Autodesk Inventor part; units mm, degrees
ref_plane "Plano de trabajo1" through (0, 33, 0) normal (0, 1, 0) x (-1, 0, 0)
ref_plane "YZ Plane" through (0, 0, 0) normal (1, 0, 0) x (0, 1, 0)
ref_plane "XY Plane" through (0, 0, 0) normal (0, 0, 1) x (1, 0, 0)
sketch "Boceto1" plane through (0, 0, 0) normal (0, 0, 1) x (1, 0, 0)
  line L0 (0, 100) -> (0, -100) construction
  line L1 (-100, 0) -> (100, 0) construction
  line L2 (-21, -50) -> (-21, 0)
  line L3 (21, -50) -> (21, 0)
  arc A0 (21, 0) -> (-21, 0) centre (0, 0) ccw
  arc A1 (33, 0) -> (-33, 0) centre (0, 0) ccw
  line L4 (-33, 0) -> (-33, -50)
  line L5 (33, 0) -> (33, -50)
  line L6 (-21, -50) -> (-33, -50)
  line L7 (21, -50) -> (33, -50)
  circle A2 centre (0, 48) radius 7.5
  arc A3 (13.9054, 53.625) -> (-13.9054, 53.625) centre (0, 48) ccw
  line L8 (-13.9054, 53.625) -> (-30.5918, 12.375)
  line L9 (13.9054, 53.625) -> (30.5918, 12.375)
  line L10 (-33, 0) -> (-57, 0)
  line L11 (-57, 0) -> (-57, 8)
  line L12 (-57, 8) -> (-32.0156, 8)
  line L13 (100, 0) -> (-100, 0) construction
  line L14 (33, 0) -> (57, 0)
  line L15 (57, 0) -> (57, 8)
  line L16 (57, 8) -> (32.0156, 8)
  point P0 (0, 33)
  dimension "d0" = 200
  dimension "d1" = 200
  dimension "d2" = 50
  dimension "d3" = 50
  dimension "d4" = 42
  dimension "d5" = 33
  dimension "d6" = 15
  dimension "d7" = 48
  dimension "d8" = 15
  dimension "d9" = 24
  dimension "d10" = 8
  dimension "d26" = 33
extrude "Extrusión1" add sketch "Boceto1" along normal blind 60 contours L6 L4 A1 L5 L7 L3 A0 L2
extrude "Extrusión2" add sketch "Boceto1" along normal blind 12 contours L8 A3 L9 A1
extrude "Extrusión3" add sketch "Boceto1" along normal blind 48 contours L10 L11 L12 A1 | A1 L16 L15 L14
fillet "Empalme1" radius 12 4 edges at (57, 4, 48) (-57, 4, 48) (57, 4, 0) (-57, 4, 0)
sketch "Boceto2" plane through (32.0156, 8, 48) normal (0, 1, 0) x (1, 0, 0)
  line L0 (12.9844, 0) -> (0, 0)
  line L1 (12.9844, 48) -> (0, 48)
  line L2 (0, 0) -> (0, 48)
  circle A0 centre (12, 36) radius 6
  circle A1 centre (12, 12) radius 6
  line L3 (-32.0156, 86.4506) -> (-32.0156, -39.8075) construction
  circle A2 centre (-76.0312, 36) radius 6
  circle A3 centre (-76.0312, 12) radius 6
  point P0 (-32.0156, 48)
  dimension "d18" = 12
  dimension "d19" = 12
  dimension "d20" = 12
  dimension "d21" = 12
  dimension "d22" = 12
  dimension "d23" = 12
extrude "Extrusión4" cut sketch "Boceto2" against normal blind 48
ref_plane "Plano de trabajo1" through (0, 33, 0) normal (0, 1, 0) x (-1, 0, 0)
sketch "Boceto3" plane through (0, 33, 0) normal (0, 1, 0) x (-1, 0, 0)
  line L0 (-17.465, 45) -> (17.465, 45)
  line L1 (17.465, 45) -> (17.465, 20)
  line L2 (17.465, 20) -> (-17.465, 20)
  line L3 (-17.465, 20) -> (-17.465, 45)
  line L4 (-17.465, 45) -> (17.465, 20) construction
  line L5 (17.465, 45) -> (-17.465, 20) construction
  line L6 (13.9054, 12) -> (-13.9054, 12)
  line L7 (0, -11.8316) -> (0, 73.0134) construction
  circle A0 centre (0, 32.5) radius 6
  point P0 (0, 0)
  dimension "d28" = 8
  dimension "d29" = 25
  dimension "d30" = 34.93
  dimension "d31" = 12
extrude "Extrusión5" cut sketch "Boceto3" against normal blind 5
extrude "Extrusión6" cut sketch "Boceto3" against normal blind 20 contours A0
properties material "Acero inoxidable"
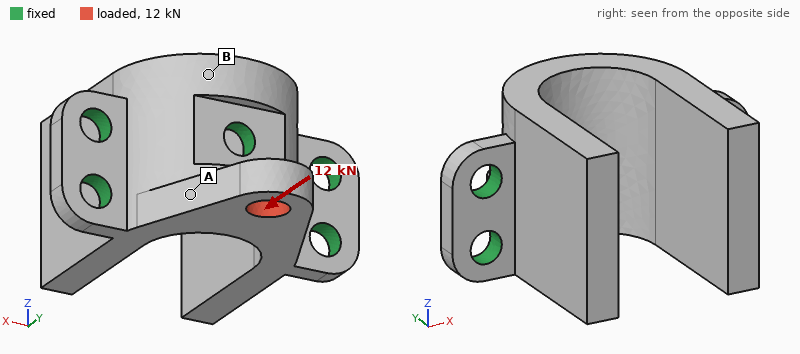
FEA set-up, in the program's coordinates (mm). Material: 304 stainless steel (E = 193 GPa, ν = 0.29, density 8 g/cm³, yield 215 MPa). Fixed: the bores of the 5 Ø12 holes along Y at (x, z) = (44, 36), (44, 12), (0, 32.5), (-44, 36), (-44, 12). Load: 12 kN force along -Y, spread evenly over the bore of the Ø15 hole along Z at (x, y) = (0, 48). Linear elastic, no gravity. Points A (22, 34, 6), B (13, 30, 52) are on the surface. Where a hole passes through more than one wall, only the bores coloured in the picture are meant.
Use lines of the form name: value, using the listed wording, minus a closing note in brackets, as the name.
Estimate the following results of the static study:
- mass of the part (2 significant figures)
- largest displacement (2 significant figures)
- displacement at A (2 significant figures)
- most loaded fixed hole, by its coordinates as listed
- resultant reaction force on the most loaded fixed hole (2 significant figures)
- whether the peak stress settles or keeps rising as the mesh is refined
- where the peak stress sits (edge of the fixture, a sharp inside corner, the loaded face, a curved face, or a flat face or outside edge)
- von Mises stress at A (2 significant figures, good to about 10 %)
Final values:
mass of the part: 1.2 kg
largest displacement: 30 µm
displacement at A: 13 µm
most loaded fixed hole, by its coordinates as listed: (0, 32.5)
resultant reaction force on the most loaded fixed hole: 6.9 kN
whether the peak stress settles or keeps rising as the mesh is refined: keeps rising
where the peak stress sits: edge of the fixture
von Mises stress at A: 31 MPa
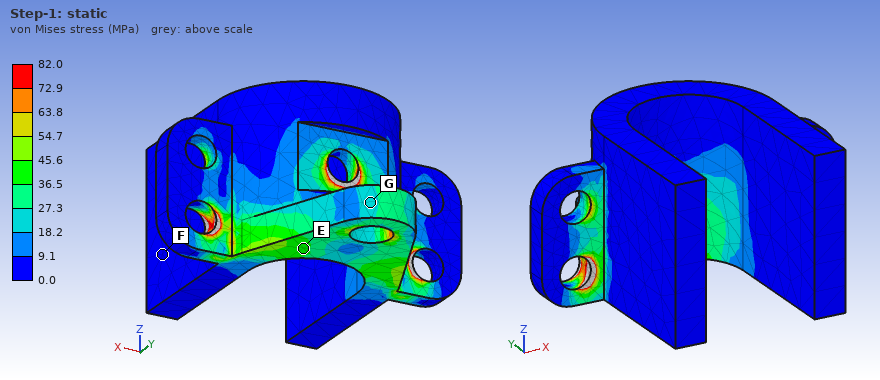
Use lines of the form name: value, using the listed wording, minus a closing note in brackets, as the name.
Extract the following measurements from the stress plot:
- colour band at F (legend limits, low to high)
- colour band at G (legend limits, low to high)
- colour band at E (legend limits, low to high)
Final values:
colour band at F: 0.0 to 9.1 MPa
colour band at G: 18.2 to 27.3 MPa
colour band at E: 36.5 to 45.6 MPa
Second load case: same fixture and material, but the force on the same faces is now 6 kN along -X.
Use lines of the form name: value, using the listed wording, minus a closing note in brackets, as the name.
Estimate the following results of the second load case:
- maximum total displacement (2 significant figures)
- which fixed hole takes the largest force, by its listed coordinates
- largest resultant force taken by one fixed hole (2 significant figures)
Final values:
maximum total displacement: 21 µm
which fixed hole takes the largest force, by its listed coordinates: (0, 32.5)
largest resultant force taken by one fixed hole: 3.1 kN
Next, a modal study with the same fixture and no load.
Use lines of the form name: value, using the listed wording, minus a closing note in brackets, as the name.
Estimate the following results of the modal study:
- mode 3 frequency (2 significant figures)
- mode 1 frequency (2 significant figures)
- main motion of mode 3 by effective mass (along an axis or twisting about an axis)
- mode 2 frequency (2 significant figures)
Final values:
mode 3 frequency: 4400 Hz
mode 1 frequency: 2700 Hz
main motion of mode 3 by effective mass: along Z
mode 2 frequency: 2700 Hz
